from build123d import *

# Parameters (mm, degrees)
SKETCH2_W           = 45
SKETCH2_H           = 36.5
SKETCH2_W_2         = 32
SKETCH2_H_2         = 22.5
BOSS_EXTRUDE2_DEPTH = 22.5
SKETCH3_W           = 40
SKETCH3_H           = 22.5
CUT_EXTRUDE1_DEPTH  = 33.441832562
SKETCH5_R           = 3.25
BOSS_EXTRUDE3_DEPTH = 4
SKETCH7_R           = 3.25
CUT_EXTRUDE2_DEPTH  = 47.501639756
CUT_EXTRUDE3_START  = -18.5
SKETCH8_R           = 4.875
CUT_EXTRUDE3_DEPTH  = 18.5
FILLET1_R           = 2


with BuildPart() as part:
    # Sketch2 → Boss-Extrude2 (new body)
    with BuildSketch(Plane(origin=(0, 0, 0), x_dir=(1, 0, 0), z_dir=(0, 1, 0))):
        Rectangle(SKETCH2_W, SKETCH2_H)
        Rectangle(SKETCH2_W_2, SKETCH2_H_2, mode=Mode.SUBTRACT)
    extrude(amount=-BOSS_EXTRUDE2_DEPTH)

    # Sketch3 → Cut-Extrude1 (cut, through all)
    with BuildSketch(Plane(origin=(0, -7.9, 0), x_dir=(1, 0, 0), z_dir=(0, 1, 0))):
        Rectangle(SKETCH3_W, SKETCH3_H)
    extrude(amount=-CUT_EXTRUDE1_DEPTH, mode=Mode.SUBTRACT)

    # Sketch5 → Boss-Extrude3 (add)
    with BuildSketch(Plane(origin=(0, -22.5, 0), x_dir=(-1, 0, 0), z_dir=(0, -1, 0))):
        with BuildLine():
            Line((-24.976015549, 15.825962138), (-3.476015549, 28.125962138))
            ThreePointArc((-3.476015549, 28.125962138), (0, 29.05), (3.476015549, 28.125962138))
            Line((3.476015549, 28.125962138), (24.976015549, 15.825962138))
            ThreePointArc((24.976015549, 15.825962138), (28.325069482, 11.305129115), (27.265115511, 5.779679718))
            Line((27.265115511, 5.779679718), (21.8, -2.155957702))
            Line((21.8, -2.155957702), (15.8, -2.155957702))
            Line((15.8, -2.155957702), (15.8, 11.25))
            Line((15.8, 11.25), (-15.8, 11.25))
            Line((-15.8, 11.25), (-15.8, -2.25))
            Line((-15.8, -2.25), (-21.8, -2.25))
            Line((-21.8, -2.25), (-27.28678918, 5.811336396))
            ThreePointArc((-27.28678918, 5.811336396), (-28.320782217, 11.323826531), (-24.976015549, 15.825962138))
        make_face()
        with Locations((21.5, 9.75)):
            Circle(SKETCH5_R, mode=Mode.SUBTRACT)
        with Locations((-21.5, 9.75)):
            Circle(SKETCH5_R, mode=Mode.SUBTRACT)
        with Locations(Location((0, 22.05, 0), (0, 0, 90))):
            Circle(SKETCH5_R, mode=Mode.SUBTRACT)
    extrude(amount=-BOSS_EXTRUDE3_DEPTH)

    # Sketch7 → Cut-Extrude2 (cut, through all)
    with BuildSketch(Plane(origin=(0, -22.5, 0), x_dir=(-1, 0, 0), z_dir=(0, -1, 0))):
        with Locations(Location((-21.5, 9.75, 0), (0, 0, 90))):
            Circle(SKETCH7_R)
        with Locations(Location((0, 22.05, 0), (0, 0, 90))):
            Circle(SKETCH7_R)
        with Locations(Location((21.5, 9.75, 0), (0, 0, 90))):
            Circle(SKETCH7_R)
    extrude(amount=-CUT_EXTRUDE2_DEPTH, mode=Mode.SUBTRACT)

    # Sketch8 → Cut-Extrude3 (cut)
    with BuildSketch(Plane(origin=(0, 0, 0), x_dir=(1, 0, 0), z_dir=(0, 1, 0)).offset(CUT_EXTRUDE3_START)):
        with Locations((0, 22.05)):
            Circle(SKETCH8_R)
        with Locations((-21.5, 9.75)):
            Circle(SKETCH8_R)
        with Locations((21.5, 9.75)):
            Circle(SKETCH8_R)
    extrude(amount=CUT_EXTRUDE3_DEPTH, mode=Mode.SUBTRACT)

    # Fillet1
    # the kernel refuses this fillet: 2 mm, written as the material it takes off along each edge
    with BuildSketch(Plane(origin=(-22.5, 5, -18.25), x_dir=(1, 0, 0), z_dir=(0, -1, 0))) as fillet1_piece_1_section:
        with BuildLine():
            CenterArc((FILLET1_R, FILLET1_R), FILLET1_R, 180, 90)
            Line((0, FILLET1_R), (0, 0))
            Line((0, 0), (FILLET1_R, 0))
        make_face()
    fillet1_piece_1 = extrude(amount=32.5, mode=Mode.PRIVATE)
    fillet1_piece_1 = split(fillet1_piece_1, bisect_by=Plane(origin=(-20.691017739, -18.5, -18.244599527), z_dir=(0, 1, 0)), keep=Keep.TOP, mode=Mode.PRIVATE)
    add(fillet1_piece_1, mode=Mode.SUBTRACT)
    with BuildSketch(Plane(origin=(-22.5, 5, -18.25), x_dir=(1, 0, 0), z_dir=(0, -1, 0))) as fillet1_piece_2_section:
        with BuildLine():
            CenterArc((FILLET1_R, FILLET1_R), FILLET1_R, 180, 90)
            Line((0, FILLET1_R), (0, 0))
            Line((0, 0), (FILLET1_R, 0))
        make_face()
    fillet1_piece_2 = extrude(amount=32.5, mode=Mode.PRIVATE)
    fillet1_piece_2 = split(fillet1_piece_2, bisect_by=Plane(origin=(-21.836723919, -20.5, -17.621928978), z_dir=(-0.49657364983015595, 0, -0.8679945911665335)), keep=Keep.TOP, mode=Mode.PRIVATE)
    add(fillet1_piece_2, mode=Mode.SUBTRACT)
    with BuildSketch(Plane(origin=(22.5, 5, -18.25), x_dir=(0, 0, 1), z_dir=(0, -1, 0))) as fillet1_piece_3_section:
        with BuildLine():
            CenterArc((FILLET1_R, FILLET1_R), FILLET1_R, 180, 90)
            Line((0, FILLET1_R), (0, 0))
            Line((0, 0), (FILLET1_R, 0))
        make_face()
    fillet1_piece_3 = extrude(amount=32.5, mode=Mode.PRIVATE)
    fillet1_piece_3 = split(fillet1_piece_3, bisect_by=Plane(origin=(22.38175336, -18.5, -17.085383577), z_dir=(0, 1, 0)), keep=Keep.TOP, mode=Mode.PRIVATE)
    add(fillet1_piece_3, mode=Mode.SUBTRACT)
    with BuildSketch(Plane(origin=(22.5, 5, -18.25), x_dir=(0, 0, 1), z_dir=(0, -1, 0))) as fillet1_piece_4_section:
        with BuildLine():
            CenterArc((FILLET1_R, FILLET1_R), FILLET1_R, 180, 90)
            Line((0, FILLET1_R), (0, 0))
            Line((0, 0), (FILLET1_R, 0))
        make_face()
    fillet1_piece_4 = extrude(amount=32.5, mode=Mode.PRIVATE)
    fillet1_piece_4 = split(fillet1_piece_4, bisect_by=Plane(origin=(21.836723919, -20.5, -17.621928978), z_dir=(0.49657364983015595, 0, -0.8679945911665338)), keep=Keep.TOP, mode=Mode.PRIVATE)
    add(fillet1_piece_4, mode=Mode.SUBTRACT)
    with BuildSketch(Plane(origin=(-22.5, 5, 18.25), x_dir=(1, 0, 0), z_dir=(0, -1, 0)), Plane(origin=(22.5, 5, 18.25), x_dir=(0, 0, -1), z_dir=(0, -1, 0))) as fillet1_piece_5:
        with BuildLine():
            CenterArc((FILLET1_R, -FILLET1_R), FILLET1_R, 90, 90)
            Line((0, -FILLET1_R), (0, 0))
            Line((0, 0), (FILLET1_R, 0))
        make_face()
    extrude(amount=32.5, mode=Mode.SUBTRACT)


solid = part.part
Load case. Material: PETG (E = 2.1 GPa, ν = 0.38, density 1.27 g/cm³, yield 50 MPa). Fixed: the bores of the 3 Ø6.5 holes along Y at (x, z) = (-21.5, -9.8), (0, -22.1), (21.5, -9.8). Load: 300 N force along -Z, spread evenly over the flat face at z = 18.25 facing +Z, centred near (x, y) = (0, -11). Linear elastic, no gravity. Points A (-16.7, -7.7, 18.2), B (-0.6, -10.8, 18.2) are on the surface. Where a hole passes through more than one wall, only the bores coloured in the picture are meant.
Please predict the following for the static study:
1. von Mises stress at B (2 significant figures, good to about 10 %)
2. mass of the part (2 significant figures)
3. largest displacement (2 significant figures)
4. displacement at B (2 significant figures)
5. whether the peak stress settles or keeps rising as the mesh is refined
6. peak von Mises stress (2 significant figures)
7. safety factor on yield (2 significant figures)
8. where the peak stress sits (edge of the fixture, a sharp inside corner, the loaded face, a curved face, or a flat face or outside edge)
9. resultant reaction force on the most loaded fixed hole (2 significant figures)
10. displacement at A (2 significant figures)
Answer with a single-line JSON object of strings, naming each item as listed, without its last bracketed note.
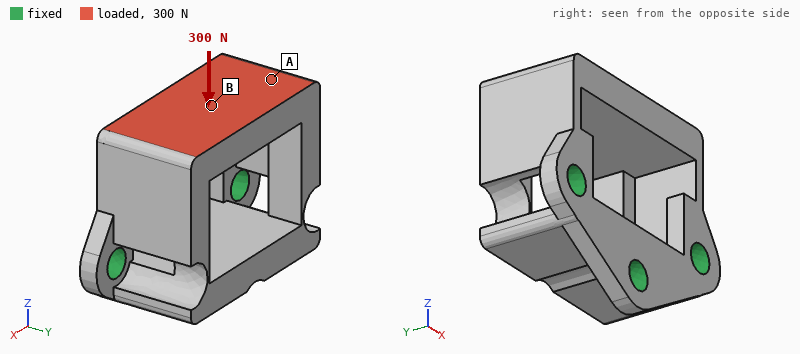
{"von Mises stress at B": "5.5 MPa", "mass of the part": "23 g", "largest displacement": "0.49 mm", "displacement at B": "0.39 mm", "whether the peak stress settles or keeps rising as the mesh is refined": "settles", "peak von Mises stress": "31 MPa", "safety factor on yield": "1.6", "where the peak stress sits": "a curved face", "resultant reaction force on the most loaded fixed hole": "150 N", "displacement at A": "0.35 mm"}
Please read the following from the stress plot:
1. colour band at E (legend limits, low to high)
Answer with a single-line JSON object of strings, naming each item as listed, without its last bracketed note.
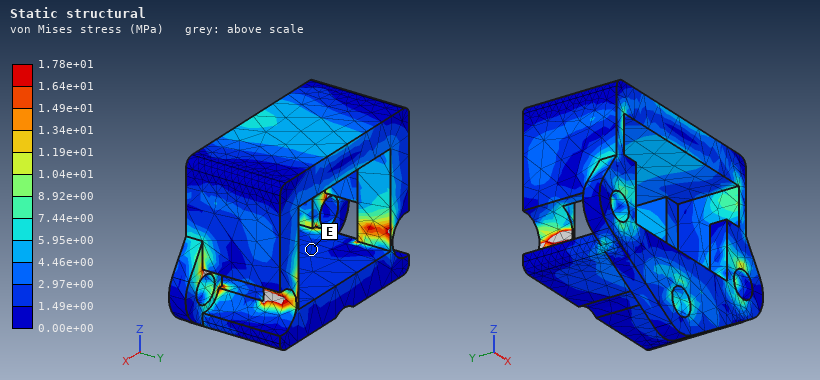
{"colour band at E": "1.49e+00 to 2.97e+00 MPa"}
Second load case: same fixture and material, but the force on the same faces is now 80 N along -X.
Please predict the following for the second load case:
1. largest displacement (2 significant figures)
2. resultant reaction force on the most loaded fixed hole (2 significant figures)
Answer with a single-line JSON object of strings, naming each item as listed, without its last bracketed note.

{"largest displacement": "0.24 mm", "resultant reaction force on the most loaded fixed hole": "53 N"}
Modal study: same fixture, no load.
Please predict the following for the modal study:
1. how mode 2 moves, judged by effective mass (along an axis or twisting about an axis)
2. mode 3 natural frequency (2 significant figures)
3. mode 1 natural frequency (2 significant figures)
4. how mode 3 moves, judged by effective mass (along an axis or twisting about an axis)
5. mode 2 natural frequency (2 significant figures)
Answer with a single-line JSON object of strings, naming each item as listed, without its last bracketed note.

{"how mode 2 moves, judged by effective mass": "along X", "mode 3 natural frequency": "1800 Hz", "mode 1 natural frequency": "870 Hz", "how mode 3 moves, judged by effective mass": "twisting about Z", "mode 2 natural frequency": "950 Hz"}
